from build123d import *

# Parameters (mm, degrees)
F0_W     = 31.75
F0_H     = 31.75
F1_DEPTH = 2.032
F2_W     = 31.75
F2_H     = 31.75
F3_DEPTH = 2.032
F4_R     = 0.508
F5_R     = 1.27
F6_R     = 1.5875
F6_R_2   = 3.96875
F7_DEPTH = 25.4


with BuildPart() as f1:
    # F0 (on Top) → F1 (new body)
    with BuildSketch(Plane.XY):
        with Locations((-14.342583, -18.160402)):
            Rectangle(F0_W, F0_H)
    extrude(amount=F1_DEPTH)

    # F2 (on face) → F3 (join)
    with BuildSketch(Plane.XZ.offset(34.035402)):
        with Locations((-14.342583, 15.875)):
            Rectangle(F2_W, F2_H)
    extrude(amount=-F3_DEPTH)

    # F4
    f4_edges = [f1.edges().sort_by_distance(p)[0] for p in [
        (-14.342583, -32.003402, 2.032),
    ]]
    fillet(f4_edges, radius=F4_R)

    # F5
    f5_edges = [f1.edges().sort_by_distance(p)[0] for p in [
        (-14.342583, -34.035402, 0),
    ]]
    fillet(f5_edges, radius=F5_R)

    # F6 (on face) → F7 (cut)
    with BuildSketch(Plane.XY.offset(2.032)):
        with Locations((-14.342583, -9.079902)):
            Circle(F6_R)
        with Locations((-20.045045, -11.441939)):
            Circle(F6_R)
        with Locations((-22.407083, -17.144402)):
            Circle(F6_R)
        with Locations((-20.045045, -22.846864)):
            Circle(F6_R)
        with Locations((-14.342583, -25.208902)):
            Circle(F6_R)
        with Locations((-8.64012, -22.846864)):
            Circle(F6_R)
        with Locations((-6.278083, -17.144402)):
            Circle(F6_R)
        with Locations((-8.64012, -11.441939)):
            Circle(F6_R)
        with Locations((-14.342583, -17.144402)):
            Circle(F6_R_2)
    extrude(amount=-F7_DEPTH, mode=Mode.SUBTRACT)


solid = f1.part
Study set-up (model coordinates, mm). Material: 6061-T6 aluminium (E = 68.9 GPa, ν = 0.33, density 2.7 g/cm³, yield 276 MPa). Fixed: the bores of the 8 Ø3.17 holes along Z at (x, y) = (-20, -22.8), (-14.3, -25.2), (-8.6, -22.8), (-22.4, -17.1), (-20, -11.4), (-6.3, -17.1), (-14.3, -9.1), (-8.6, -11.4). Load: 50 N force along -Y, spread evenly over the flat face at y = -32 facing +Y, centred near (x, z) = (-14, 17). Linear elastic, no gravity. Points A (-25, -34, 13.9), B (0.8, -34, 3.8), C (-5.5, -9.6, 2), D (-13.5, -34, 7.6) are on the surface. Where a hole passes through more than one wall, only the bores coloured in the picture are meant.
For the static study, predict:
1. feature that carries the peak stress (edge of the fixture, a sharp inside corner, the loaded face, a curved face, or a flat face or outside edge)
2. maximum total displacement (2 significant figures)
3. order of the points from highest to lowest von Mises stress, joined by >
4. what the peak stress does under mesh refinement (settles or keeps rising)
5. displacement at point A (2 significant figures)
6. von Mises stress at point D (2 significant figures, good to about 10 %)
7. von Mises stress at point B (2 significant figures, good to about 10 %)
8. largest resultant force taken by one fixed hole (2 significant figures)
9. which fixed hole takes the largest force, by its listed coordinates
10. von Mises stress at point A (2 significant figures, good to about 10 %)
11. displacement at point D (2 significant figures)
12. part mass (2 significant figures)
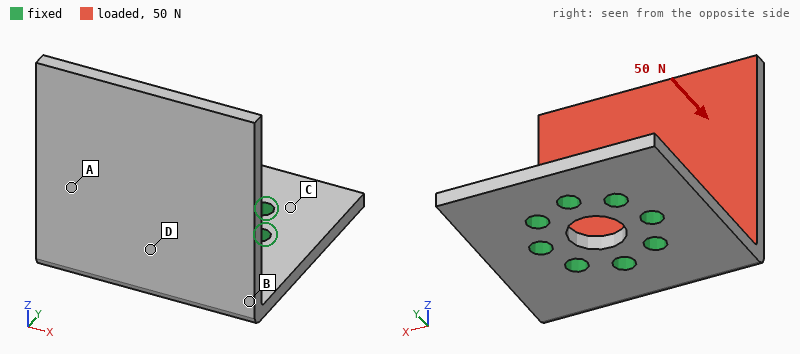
edge of the fixture
0.23 mm
B > D > A > C
keeps rising
0.080 mm
21 MPa
30 MPa
55 N
(-14.3, -25.2)
12 MPa
0.041 mm
10 g
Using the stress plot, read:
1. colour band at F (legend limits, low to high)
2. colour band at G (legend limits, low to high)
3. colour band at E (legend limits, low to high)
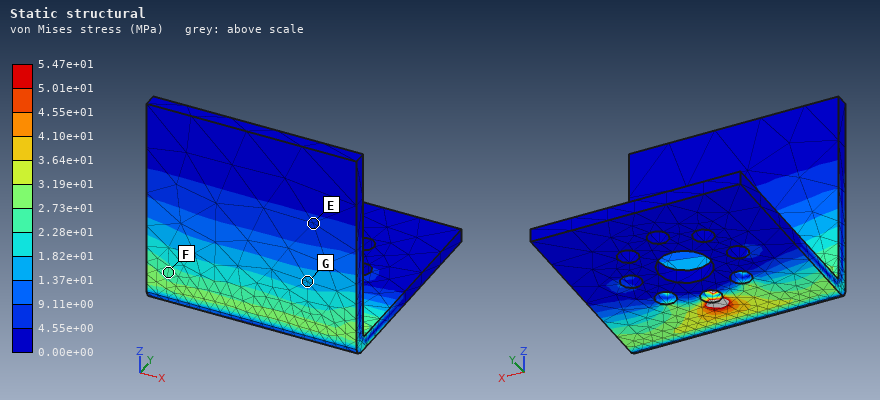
2.28e+01 to 2.73e+01 MPa
1.37e+01 to 1.82e+01 MPa
4.55e+00 to 9.11e+00 MPa
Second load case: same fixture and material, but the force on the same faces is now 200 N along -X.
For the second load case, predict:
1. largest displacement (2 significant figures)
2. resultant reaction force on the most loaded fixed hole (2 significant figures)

0.19 mm
190 N
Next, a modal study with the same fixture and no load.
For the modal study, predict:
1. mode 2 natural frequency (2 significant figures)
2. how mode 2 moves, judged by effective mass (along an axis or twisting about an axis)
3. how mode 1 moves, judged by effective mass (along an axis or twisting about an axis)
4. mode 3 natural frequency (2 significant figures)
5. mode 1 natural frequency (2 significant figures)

2600 Hz
along X
along Y
4100 Hz
1300 Hz
